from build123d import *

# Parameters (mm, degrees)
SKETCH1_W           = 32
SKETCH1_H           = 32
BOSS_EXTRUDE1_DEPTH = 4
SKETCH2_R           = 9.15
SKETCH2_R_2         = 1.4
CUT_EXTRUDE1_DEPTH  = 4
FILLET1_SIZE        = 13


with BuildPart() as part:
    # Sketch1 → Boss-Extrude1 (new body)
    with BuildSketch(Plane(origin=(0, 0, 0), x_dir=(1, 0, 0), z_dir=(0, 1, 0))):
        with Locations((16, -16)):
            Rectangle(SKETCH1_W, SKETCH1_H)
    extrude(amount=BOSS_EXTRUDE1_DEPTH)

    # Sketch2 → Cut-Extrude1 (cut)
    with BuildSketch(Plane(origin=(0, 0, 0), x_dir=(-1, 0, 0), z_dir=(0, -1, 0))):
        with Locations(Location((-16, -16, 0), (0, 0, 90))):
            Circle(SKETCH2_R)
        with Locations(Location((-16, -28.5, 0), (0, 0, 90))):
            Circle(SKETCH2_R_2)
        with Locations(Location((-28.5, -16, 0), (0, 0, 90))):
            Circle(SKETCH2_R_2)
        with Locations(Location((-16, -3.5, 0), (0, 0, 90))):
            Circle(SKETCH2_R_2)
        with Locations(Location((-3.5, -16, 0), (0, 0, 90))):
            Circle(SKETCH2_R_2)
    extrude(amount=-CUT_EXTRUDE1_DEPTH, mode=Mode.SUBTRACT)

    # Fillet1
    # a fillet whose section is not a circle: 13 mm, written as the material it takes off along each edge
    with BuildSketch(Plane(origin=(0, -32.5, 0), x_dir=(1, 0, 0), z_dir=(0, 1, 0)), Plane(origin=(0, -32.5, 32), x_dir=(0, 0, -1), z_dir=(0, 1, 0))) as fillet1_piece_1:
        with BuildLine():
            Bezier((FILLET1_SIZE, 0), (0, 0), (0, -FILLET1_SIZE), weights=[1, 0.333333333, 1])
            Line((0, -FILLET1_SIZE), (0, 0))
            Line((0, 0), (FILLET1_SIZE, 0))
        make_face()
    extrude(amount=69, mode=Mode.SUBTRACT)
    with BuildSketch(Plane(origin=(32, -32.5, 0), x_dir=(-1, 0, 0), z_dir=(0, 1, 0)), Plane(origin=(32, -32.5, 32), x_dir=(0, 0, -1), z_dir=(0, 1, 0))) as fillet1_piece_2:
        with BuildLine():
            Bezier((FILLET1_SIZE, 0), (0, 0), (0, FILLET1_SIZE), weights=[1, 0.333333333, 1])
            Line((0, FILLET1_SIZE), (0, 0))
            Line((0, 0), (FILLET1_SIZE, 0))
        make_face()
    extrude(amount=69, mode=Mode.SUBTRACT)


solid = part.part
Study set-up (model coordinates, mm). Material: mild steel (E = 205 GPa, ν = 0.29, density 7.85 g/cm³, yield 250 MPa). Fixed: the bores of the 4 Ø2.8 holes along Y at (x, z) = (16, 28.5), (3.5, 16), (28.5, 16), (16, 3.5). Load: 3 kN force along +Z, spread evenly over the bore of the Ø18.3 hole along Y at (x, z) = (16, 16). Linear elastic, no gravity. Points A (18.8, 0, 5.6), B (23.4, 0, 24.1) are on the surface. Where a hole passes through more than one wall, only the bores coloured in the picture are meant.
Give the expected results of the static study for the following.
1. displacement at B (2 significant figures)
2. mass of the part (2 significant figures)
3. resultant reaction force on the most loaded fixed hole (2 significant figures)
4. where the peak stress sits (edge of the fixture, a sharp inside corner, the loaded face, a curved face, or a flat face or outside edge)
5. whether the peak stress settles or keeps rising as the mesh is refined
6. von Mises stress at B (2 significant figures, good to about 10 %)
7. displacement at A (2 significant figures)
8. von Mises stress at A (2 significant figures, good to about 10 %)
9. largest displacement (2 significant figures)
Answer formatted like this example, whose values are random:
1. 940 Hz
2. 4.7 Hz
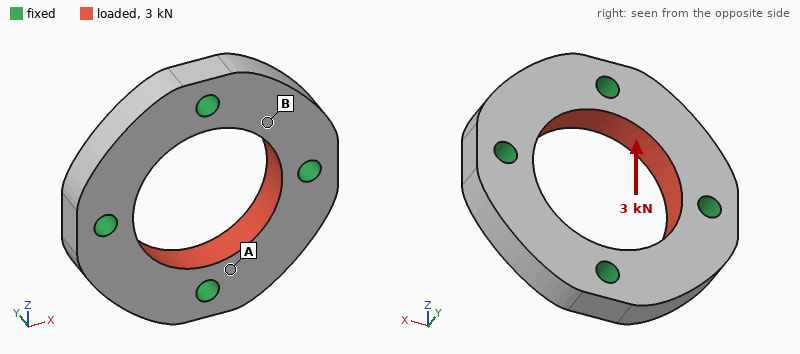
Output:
1. 1.0 µm
2. 16 g
3. 860 N
4. edge of the fixture
5. keeps rising
6. 11 MPa
7. 0.48 µm
8. 23 MPa
9. 1.1 µm
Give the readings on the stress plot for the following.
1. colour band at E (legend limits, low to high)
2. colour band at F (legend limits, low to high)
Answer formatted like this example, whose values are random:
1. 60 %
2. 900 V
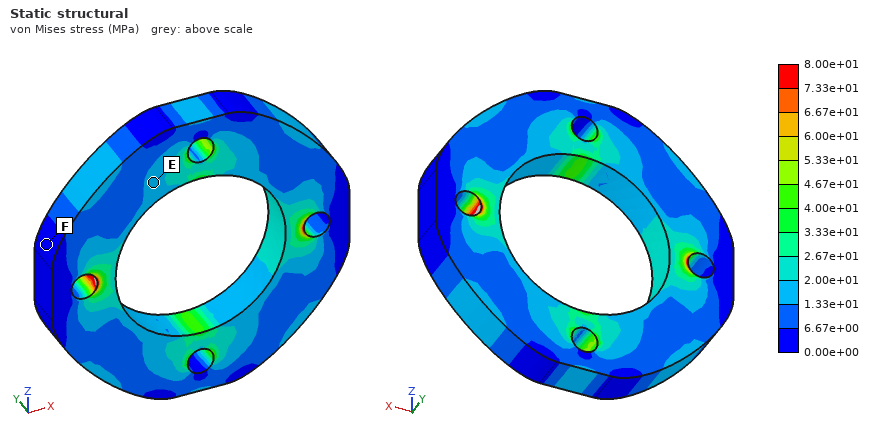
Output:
1. 1.33e+01 to 2.00e+01 MPa
2. 0.00e+00 to 6.67e+00 MPa
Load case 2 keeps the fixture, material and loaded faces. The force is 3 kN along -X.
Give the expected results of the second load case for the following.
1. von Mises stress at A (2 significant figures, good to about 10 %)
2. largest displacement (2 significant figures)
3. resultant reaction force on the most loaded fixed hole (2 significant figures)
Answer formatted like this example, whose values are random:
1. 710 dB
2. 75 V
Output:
1. 22 MPa
2. 1.1 µm
3. 860 N
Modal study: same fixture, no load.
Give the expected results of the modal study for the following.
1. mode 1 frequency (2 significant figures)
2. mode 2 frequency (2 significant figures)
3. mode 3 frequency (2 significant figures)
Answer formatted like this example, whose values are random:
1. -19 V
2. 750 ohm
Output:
1. 42 kHz
2. 44 kHz
3. 44 kHz
